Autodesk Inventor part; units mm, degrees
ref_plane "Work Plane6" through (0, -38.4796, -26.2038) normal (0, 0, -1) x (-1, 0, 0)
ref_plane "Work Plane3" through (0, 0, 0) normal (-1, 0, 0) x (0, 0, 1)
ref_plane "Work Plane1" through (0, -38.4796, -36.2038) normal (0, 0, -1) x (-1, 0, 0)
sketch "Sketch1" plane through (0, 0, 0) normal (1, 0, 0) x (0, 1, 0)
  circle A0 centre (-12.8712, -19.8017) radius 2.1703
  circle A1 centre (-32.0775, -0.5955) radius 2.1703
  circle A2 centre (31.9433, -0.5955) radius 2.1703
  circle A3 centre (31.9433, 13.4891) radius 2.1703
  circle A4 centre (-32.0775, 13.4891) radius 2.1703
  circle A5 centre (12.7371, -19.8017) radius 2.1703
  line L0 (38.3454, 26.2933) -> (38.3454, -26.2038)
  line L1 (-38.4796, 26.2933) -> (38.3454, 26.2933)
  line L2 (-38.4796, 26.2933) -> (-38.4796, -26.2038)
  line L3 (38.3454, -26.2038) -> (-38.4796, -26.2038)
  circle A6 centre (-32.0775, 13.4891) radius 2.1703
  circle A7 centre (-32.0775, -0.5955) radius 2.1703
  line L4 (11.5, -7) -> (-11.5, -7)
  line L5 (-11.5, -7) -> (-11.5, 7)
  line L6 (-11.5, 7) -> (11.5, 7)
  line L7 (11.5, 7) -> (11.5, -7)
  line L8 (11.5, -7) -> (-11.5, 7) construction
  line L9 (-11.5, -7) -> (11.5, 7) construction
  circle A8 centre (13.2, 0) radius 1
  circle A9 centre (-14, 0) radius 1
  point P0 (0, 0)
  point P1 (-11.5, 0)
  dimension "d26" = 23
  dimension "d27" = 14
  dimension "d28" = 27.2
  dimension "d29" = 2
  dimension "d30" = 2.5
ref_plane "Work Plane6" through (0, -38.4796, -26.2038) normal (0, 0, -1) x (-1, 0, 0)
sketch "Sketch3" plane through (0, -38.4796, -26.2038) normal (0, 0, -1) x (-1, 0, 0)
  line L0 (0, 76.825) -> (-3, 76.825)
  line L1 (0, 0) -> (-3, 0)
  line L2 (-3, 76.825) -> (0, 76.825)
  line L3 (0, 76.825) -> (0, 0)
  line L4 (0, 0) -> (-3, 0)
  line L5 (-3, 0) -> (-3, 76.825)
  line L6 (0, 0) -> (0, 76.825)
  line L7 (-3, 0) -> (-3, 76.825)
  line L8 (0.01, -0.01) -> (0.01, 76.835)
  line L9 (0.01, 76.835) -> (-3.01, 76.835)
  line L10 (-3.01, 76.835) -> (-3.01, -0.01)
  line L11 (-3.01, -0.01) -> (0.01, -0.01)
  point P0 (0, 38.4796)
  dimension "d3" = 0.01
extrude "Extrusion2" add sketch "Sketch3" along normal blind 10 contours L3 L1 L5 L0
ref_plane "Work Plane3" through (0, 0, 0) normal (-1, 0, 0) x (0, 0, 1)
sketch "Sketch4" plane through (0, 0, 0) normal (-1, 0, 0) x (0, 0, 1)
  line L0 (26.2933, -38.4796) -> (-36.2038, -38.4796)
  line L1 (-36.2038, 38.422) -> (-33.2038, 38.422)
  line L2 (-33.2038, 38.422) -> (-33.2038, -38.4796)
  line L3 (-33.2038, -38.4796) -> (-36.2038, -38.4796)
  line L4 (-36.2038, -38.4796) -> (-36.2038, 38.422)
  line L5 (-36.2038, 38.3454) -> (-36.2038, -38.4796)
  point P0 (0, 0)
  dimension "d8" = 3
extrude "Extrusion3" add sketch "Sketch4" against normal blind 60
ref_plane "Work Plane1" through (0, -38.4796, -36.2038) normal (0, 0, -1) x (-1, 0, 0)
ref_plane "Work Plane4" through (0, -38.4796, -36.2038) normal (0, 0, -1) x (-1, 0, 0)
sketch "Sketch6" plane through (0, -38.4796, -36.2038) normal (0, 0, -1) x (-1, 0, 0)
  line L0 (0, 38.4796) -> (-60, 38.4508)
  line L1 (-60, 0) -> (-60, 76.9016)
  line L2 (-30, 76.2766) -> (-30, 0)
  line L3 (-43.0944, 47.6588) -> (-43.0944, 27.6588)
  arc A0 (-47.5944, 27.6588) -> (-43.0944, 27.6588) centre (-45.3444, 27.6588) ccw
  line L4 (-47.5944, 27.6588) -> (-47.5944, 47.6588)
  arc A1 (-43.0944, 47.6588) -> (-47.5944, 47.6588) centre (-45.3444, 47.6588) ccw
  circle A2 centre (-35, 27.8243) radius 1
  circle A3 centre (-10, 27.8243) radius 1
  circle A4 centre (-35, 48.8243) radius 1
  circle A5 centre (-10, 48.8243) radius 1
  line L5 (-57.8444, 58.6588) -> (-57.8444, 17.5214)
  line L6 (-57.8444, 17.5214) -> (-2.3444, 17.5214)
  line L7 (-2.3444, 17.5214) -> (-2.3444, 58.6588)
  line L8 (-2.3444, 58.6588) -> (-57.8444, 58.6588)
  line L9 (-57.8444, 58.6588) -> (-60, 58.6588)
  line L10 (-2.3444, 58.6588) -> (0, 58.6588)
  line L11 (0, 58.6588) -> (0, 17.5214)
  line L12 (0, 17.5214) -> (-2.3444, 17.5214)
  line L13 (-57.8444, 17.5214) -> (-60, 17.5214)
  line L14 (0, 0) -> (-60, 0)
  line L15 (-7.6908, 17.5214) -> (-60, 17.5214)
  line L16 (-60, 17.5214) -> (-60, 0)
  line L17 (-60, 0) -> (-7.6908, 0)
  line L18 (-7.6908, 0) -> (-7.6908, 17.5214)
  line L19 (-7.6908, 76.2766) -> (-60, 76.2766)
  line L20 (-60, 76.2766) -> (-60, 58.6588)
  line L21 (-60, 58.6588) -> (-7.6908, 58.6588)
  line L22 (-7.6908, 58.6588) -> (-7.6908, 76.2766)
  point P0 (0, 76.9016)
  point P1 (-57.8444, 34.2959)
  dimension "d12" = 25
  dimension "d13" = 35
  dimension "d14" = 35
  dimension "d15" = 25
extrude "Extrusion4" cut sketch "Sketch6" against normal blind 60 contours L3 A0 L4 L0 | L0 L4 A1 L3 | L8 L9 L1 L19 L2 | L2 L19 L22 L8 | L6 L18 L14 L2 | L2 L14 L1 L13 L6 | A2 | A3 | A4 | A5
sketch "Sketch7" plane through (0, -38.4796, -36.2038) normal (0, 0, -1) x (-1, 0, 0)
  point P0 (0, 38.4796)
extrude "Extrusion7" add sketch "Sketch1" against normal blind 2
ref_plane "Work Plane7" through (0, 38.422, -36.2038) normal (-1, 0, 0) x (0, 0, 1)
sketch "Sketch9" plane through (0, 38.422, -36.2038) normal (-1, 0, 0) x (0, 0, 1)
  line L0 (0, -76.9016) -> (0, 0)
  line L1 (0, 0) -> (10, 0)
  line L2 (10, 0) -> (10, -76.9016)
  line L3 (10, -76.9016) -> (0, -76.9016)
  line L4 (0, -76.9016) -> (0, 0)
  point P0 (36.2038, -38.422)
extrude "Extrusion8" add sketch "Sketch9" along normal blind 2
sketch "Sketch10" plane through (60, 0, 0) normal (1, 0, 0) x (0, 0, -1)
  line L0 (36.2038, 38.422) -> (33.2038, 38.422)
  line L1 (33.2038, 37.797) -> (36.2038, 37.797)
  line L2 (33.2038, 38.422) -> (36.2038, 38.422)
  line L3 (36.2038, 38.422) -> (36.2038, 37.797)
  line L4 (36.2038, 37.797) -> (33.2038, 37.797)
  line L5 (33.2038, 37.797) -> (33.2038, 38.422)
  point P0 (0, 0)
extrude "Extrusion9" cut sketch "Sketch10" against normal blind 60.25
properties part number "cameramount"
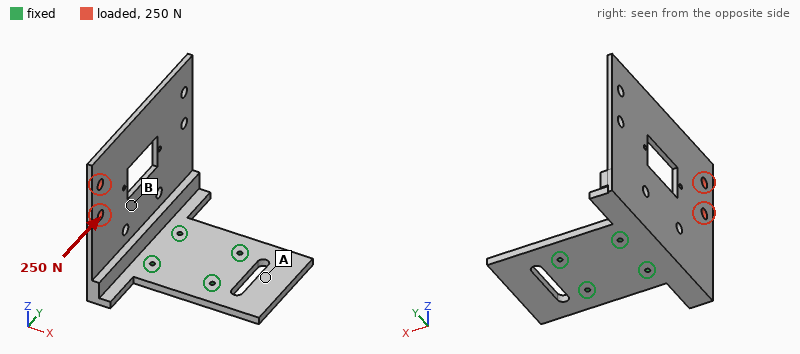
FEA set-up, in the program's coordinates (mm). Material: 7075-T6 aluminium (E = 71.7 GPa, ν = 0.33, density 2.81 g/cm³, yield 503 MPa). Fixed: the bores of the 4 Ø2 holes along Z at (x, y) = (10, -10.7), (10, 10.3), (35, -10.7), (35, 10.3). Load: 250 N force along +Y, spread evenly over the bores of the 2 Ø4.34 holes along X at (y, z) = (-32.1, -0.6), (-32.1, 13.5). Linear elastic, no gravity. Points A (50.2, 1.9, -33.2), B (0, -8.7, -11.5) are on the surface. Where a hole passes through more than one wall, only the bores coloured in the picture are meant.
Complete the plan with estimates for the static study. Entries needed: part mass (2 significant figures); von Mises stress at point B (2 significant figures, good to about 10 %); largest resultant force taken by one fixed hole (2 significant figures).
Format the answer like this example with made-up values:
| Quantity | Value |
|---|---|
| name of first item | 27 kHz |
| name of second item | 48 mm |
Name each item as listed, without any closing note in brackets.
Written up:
| Quantity | Value |
|---|---|
| part mass | 51 g |
| von Mises stress at point B | 9.2 MPa |
| largest resultant force taken by one fixed hole | 470 N |
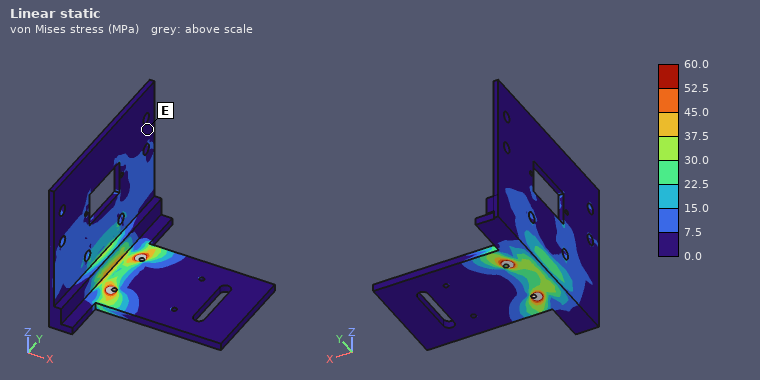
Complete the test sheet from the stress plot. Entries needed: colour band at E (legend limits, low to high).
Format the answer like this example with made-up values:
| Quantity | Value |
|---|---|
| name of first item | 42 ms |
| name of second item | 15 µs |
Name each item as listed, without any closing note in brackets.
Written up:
| Quantity | Value |
|---|---|
| colour band at E | 0.0 to 7.5 MPa |
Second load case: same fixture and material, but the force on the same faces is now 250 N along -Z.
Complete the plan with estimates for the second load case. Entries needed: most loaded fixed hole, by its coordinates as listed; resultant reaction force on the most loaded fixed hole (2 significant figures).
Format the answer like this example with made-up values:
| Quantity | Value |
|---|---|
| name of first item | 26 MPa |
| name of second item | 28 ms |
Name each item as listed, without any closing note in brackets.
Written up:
| Quantity | Value |
|---|---|
| most loaded fixed hole, by its coordinates as listed | (10, -10.7) |
| resultant reaction force on the most loaded fixed hole | 490 N |
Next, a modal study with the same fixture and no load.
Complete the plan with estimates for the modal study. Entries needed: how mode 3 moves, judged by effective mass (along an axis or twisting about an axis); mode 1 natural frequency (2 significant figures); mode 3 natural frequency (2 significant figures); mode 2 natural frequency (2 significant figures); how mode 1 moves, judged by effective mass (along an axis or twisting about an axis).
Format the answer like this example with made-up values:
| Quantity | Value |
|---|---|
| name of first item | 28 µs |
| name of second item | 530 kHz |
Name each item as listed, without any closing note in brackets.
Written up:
| Quantity | Value |
|---|---|
| how mode 3 moves, judged by effective mass | along Y |
| mode 1 natural frequency | 450 Hz |
| mode 3 natural frequency | 1600 Hz |
| mode 2 natural frequency | 920 Hz |
| how mode 1 moves, judged by effective mass | along X |
